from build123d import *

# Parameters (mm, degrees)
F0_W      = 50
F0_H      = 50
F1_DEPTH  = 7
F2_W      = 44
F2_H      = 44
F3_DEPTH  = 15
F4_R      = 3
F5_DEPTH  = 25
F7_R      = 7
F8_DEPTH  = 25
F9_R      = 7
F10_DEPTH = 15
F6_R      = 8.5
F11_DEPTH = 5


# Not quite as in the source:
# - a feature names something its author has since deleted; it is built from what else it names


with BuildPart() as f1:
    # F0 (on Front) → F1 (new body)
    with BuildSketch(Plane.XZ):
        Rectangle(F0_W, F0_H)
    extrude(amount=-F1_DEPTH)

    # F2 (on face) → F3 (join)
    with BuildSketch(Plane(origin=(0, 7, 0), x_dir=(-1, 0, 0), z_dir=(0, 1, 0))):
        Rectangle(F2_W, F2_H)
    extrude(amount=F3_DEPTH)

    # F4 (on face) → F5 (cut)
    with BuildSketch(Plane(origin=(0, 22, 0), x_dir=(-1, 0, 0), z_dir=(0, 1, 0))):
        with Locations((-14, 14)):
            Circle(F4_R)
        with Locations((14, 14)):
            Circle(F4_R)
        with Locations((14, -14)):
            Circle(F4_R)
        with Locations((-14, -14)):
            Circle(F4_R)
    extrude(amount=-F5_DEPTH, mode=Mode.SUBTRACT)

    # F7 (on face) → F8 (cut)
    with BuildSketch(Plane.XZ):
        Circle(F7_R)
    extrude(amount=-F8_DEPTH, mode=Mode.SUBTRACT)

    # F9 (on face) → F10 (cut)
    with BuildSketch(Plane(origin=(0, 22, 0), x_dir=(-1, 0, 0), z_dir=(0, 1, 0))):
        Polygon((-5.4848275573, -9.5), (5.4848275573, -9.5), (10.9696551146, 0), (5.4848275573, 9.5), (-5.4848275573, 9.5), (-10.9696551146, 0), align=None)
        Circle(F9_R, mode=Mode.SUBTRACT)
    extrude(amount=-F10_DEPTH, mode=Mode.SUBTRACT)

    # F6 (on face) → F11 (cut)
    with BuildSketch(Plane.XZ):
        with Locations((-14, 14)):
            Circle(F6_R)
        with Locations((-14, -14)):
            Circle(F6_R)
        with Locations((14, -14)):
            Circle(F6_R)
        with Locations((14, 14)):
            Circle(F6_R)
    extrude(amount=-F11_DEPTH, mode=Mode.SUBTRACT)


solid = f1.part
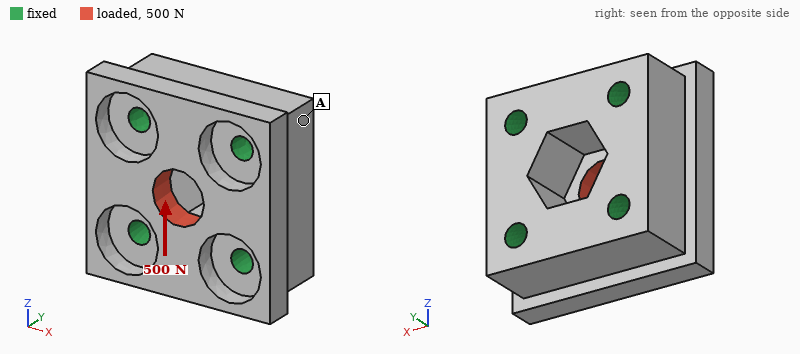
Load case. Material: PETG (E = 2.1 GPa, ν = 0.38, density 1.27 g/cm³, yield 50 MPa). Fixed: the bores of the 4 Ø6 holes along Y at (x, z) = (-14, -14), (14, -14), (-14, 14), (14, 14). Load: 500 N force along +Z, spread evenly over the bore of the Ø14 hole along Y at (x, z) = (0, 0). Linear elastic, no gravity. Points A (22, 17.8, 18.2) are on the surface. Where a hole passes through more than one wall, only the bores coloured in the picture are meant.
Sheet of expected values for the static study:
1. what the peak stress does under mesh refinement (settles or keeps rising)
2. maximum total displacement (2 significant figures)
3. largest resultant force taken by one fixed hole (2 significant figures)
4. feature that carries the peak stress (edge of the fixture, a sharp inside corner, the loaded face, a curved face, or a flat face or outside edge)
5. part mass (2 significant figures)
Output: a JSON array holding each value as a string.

["keeps rising", "22 µm", "140 N", "edge of the fixture", "44 g"]
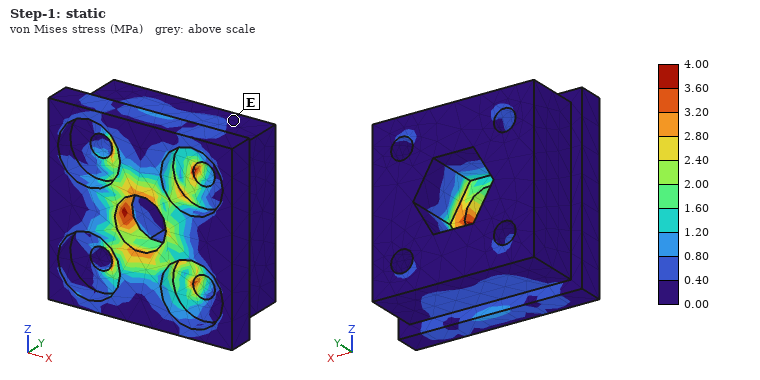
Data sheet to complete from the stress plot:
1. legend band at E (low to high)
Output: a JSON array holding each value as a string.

["0.00 to 0.40 MPa"]
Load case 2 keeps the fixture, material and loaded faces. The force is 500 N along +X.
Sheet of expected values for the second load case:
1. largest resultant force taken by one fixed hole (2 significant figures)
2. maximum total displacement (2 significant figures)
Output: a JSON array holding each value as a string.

["140 N", "22 µm"]
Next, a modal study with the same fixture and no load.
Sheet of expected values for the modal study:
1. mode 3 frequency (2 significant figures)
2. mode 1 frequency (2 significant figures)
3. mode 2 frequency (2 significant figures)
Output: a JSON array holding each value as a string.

["9400 Hz", "8600 Hz", "9400 Hz"]
